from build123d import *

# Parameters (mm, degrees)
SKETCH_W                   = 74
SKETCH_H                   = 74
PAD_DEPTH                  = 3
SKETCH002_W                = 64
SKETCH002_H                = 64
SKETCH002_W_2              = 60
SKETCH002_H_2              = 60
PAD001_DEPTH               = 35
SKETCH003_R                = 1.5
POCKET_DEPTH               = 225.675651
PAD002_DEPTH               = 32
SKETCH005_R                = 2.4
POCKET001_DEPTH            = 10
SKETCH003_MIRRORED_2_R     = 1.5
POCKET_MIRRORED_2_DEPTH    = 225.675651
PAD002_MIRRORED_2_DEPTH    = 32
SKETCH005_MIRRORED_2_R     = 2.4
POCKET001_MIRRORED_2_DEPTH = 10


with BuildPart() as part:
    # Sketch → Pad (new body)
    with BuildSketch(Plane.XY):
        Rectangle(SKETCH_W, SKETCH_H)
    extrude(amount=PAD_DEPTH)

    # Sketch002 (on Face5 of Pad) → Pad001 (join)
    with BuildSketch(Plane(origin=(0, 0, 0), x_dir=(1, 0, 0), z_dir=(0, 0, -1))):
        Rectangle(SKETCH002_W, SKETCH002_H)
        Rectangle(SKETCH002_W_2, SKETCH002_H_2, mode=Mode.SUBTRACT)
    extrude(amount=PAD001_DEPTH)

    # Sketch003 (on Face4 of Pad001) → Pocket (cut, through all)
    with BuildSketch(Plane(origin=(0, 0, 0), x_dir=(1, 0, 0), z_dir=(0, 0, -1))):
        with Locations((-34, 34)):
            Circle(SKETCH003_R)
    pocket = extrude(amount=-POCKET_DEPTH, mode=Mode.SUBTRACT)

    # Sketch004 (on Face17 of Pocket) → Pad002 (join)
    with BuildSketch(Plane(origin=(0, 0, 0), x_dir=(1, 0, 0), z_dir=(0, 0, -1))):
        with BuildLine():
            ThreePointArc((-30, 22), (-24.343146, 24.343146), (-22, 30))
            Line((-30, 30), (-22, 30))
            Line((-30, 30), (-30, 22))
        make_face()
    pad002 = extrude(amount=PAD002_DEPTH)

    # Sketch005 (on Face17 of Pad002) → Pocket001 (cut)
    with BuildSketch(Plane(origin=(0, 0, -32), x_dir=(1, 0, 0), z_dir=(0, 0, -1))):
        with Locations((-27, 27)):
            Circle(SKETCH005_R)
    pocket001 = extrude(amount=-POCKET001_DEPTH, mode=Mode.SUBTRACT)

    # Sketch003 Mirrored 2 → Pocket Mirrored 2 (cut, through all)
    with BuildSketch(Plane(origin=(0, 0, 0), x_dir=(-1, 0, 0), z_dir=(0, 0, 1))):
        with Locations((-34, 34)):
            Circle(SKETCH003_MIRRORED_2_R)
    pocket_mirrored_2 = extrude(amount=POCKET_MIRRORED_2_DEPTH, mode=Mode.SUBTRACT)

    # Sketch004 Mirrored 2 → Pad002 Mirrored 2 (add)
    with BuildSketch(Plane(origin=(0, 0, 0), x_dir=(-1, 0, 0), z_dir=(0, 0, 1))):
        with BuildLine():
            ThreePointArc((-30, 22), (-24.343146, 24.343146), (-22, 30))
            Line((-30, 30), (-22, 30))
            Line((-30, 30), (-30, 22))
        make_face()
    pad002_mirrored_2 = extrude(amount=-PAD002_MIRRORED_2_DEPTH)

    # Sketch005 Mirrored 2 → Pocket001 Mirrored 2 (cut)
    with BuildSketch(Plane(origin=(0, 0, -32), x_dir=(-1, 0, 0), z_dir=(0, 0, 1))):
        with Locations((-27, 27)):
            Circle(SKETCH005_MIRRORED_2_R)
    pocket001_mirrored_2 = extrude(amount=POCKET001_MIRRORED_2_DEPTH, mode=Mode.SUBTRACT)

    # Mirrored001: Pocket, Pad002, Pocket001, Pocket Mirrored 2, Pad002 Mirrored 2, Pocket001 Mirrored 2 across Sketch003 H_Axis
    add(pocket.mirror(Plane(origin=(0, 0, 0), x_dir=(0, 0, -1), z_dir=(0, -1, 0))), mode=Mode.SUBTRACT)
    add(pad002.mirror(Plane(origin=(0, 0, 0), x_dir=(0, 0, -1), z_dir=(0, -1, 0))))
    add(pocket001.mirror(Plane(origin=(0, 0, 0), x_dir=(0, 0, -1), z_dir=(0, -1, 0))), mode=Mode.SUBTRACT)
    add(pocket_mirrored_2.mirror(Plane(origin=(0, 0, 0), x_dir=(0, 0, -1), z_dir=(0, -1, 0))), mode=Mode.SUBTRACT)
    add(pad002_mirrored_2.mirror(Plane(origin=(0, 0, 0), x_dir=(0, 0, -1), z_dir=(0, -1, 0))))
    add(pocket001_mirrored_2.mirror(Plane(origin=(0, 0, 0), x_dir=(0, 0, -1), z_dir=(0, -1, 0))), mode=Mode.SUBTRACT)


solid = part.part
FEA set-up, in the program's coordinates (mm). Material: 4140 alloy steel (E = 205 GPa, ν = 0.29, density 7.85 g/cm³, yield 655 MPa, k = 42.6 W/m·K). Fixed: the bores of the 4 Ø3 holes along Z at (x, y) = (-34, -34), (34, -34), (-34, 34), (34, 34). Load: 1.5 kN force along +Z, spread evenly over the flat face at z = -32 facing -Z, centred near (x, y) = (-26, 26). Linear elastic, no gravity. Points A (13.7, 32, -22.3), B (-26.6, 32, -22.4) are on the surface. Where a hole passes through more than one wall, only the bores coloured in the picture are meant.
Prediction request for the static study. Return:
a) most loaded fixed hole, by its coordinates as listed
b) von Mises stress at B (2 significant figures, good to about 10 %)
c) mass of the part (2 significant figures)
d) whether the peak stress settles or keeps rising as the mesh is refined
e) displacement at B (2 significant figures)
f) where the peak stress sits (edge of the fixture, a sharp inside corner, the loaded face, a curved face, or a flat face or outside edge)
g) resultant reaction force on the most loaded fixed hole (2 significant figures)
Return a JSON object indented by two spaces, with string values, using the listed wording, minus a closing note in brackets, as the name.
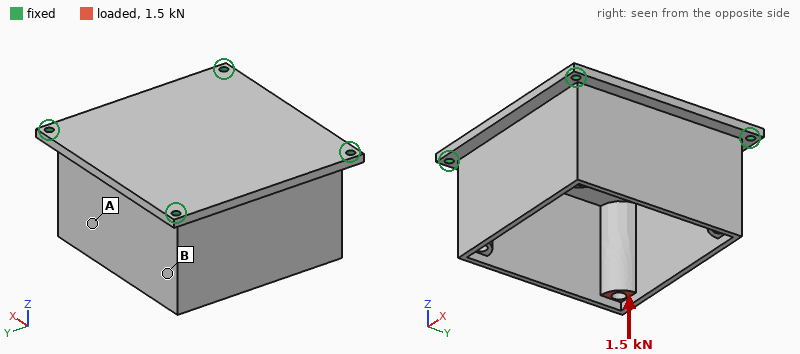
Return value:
{
  "most loaded fixed hole, by its coordinates as listed": "(-34, 34)",
  "von Mises stress at B": "13 MPa",
  "mass of the part": "310 g",
  "whether the peak stress settles or keeps rising as the mesh is refined": "keeps rising",
  "displacement at B": "9.5 µm",
  "where the peak stress sits": "edge of the fixture",
  "resultant reaction force on the most loaded fixed hole": "1.3 kN"
}
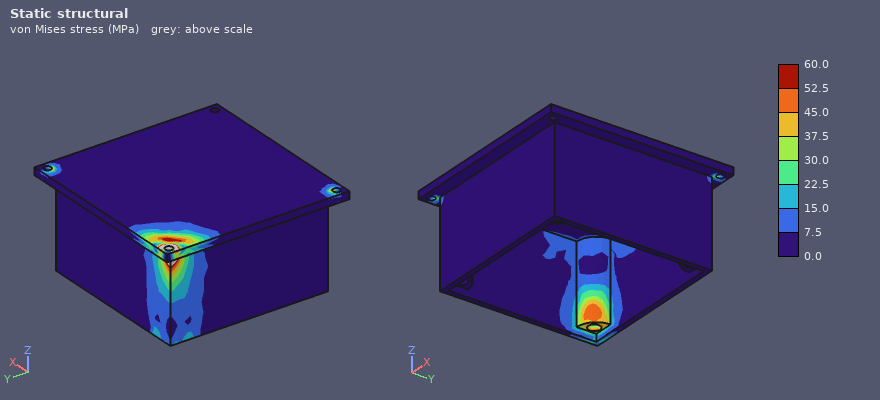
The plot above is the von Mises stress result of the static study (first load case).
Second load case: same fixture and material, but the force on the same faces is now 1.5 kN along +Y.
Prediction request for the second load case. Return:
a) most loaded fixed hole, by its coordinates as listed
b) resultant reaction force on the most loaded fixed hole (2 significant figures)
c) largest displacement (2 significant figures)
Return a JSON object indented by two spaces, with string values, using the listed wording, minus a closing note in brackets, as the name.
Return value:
{
  "most loaded fixed hole, by its coordinates as listed": "(-34, -34)",
  "resultant reaction force on the most loaded fixed hole": "1.1 kN",
  "largest displacement": "42 µm"
}
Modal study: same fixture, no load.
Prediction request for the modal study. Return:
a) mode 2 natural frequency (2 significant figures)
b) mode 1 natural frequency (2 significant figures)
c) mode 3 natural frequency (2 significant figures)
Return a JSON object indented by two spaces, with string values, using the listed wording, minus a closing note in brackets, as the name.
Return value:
{
  "mode 2 natural frequency": "4500 Hz",
  "mode 1 natural frequency": "4000 Hz",
  "mode 3 natural frequency": "4500 Hz"
}
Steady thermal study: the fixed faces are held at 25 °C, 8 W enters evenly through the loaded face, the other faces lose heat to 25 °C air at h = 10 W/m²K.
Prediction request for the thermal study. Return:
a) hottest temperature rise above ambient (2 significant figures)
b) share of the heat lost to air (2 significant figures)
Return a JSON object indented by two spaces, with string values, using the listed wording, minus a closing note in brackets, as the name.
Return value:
{
  "hottest temperature rise above ambient": "62 K",
  "share of the heat lost to air": "33 %"
}
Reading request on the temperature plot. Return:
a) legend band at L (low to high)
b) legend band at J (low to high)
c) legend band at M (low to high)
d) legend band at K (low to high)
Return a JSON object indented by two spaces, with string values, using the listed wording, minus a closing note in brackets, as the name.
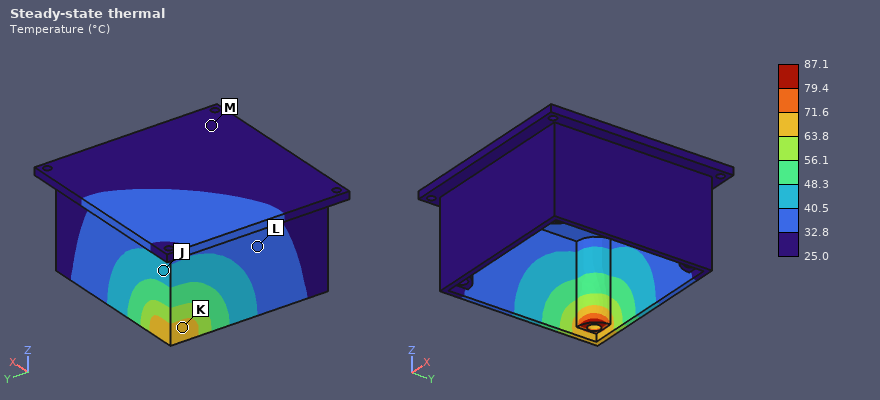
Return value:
{
  "legend band at L": "32.8 to 40.5 °C",
  "legend band at J": "40.5 to 48.3 °C",
  "legend band at M": "25.0 to 32.8 °C",
  "legend band at K": "63.8 to 71.6 °C"
}
